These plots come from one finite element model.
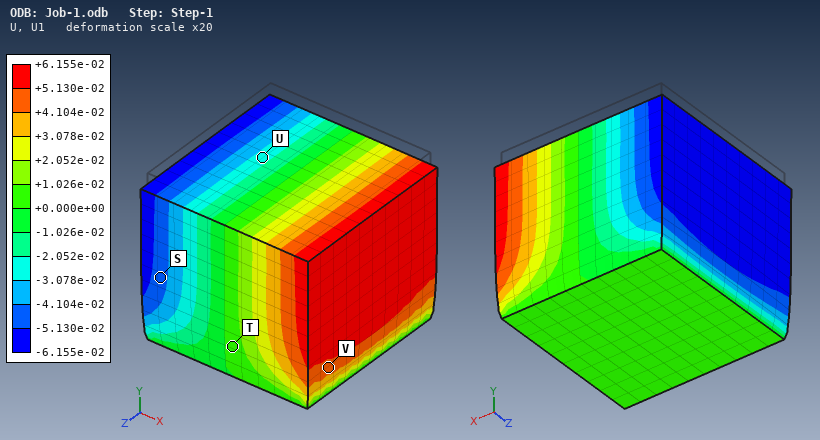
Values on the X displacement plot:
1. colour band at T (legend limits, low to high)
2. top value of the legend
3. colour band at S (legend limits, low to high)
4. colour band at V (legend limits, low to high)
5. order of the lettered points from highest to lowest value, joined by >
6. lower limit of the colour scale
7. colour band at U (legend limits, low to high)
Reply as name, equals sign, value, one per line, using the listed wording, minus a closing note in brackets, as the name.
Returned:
colour band at T = +0.000e+00 to +1.026e-02
top value of the legend = +6.155e-02
colour band at S = -5.130e-02 to -4.104e-02
colour band at V = +4.104e-02 to +5.130e-02
order of the lettered points from highest to lowest value, joined by > = V > T > U > S
lower limit of the colour scale = -6.155e-02
colour band at U = -3.078e-02 to -2.052e-02
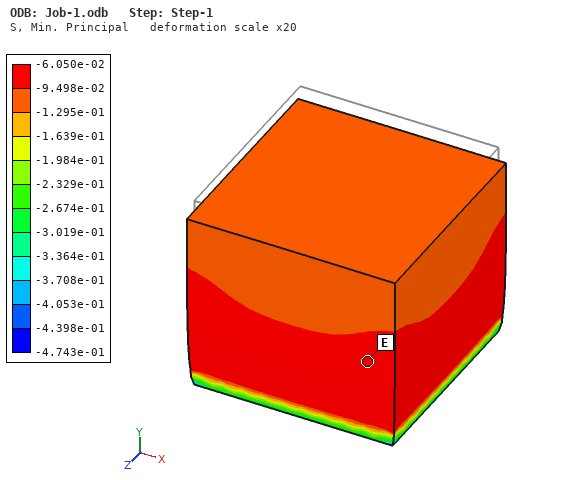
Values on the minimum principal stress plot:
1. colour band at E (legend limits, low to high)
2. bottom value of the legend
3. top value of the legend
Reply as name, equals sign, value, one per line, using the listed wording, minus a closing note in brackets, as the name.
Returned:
colour band at E = -9.498e-02 to -6.050e-02
bottom value of the legend = -4.743e-01
top value of the legend = -6.050e-02
